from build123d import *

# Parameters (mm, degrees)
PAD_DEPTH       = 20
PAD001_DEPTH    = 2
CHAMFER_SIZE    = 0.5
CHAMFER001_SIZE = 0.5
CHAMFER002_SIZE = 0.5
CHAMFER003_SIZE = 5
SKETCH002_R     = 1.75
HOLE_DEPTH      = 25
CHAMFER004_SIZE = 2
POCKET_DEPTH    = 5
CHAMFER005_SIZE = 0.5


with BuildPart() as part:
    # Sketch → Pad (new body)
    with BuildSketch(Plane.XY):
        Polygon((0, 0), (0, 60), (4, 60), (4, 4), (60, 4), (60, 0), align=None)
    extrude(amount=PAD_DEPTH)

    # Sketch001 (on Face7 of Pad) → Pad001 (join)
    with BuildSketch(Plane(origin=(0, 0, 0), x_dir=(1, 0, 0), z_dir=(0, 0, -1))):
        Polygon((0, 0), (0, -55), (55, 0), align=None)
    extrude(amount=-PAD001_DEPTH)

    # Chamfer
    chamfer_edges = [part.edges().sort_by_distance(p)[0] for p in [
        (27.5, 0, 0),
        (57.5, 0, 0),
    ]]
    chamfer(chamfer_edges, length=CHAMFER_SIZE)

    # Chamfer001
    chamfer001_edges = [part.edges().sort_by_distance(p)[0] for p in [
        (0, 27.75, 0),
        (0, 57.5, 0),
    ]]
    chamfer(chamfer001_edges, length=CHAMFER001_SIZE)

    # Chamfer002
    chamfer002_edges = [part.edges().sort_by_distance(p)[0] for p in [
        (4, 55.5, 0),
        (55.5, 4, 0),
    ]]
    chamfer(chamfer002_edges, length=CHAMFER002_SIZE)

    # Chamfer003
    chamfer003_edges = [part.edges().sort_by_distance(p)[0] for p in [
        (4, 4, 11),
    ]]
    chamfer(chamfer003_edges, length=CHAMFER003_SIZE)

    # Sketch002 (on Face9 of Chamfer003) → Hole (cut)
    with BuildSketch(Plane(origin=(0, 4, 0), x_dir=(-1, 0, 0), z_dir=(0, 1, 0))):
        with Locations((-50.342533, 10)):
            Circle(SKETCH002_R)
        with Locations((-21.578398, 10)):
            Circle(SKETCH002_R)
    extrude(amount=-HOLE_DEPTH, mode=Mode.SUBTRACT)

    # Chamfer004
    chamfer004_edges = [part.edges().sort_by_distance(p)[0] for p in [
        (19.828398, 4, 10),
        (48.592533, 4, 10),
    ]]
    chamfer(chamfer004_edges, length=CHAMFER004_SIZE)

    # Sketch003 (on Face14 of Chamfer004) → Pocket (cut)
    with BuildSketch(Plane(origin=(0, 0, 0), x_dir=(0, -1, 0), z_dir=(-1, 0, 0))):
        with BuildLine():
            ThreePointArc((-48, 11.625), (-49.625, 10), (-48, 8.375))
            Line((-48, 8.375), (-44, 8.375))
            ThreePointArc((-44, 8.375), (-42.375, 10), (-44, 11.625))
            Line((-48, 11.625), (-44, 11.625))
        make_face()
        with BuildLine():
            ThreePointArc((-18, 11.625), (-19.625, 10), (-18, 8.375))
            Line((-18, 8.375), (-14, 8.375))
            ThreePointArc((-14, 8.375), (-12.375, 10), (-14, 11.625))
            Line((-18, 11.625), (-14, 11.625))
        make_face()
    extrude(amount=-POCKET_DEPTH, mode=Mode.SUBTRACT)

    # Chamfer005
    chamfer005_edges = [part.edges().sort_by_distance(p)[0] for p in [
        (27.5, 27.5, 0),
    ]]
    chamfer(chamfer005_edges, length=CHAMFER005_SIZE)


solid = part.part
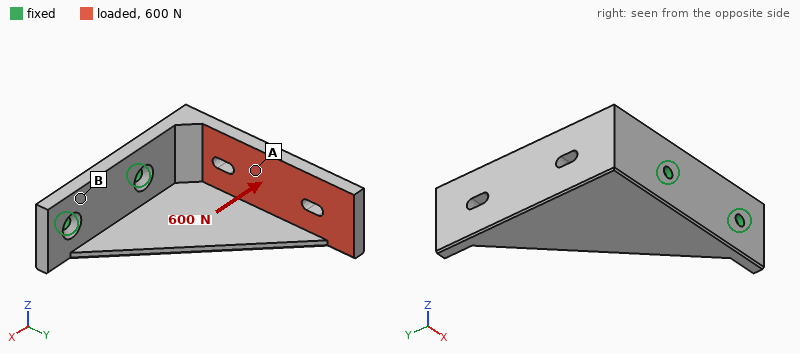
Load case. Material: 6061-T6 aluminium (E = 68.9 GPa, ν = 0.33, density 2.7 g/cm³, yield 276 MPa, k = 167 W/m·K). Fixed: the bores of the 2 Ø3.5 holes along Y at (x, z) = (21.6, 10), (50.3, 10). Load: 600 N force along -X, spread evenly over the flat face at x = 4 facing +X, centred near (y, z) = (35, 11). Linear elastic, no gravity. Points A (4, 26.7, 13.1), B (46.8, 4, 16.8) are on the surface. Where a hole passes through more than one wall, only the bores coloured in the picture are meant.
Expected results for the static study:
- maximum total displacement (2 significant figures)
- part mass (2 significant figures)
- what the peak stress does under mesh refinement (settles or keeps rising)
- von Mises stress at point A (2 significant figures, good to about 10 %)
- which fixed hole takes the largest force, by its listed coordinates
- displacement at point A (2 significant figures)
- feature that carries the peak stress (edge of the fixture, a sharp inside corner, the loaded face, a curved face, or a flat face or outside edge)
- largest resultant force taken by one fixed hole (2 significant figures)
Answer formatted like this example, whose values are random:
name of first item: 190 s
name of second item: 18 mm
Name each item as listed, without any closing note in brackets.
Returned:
maximum total displacement: 0.65 mm
part mass: 31 g
what the peak stress does under mesh refinement: keeps rising
von Mises stress at point A: 59 MPa
which fixed hole takes the largest force, by its listed coordinates: (50.3, 10)
displacement at point A: 0.23 mm
feature that carries the peak stress: edge of the fixture
largest resultant force taken by one fixed hole: 940 N
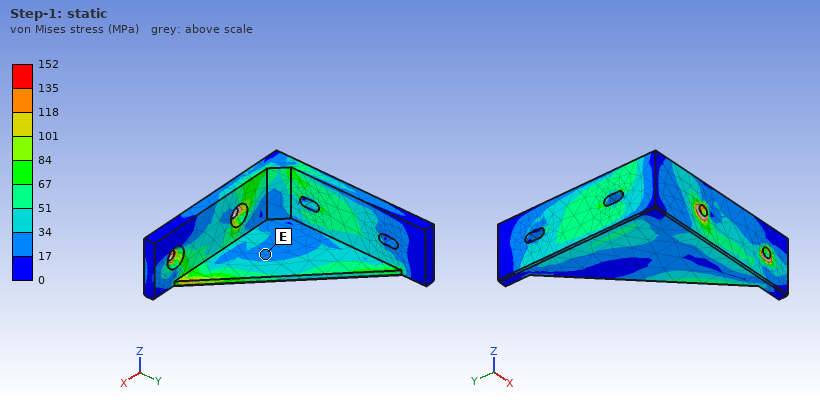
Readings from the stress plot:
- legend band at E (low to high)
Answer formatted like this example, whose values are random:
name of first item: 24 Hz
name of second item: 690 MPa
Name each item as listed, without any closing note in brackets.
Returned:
legend band at E: 17 to 34 MPa
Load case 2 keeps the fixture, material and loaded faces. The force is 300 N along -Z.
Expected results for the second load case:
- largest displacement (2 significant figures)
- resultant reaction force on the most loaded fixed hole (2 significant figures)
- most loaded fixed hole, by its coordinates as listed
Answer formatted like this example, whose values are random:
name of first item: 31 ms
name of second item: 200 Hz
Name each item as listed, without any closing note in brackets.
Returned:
largest displacement: 0.93 mm
resultant reaction force on the most loaded fixed hole: 440 N
most loaded fixed hole, by its coordinates as listed: (21.6, 10)
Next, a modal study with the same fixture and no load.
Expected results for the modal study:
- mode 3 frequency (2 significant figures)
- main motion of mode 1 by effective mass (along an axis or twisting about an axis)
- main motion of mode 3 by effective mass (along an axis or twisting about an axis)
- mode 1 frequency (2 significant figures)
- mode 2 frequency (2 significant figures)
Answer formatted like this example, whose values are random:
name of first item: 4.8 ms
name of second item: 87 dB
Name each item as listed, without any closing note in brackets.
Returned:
mode 3 frequency: 4200 Hz
main motion of mode 1 by effective mass: along Z
main motion of mode 3 by effective mass: along Y
mode 1 frequency: 970 Hz
mode 2 frequency: 2000 Hz
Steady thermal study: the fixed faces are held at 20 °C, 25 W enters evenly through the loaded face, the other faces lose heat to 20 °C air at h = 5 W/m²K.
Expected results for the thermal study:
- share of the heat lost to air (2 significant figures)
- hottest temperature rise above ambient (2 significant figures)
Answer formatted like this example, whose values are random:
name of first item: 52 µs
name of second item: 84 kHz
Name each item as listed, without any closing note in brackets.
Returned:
share of the heat lost to air: 3.5 %
hottest temperature rise above ambient: 63 K
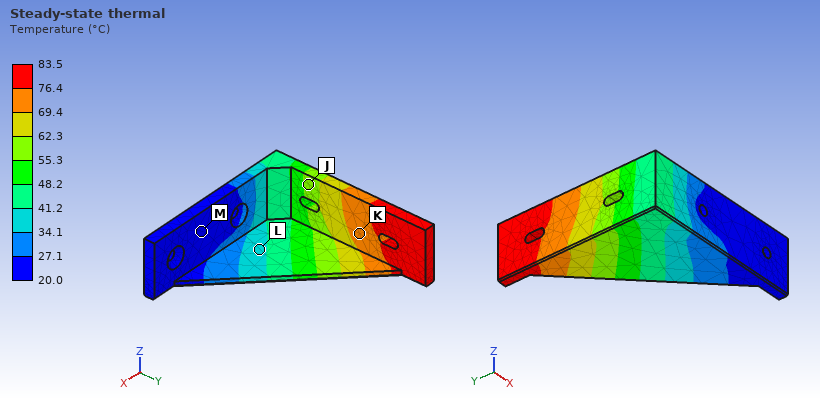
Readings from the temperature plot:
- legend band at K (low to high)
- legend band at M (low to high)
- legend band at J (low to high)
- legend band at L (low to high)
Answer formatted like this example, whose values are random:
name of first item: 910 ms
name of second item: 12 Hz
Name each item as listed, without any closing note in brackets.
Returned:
legend band at K: 69.4 to 76.4 °C
legend band at M: 20.0 to 27.1 °C
legend band at J: 55.3 to 62.3 °C
legend band at L: 34.1 to 41.2 °C
